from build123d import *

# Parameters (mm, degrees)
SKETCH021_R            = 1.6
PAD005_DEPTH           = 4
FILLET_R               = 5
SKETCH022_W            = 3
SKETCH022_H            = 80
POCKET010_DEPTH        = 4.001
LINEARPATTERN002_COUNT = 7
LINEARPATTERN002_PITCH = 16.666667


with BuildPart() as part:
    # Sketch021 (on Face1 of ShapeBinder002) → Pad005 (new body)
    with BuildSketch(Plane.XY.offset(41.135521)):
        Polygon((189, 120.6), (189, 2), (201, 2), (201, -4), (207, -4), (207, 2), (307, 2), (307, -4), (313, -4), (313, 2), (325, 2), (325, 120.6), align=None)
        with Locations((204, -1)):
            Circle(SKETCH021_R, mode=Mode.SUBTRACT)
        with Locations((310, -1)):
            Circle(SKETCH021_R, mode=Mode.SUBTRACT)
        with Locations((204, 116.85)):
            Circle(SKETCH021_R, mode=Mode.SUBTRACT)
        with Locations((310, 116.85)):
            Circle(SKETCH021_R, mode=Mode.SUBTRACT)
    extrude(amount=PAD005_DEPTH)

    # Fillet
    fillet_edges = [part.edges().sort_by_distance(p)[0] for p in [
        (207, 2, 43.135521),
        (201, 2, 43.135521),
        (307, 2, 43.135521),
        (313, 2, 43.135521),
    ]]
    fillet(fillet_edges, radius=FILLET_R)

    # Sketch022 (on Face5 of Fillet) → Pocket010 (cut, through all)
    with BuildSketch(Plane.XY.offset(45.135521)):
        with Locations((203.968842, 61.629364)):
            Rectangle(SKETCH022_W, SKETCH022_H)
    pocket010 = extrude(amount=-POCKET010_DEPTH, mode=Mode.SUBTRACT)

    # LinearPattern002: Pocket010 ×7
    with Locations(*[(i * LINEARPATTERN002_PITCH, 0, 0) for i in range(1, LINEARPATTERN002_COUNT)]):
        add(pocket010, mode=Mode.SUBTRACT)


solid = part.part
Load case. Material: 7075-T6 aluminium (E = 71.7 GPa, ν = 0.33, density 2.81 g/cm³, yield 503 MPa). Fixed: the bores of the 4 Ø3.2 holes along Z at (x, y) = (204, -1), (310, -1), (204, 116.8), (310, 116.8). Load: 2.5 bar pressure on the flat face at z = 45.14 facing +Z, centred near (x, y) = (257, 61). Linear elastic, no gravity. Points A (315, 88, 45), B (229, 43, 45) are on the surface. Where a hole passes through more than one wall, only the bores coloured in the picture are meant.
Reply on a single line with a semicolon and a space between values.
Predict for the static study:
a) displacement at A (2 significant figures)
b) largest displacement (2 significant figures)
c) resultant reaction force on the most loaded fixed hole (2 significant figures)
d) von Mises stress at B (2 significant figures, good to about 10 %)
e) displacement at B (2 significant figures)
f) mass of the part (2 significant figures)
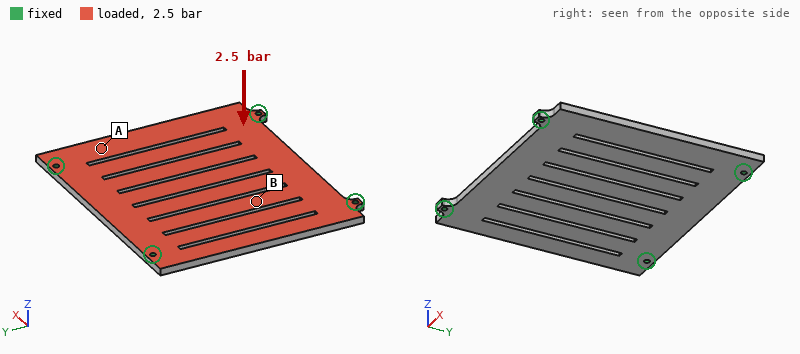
0.26 mm; 1.4 mm; 980 N; 80 MPa; 1.0 mm; 160 g
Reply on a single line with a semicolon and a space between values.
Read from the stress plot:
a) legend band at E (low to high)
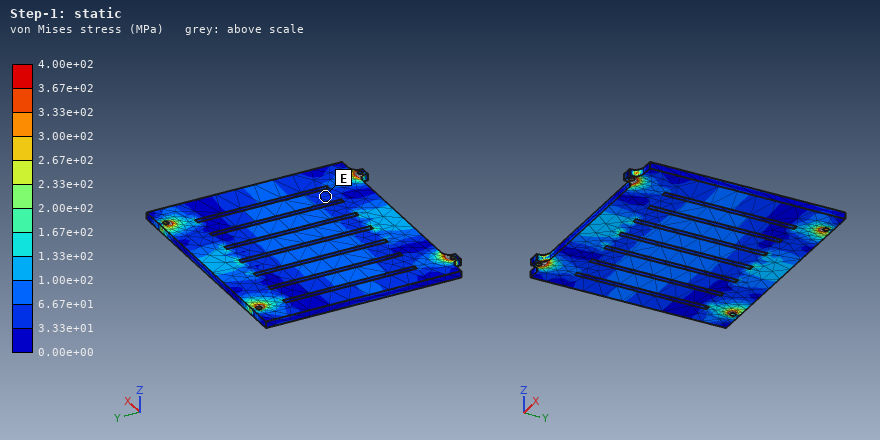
3.33e+01 to 6.67e+01 MPa
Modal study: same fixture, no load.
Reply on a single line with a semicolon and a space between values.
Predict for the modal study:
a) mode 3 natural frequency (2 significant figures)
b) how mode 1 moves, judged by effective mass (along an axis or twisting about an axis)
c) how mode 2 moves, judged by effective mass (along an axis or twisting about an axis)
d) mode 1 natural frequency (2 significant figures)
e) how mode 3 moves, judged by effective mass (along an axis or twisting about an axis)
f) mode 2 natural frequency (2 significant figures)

1400 Hz; along Z; twisting about Y; 780 Hz; along Z; 1300 Hz
